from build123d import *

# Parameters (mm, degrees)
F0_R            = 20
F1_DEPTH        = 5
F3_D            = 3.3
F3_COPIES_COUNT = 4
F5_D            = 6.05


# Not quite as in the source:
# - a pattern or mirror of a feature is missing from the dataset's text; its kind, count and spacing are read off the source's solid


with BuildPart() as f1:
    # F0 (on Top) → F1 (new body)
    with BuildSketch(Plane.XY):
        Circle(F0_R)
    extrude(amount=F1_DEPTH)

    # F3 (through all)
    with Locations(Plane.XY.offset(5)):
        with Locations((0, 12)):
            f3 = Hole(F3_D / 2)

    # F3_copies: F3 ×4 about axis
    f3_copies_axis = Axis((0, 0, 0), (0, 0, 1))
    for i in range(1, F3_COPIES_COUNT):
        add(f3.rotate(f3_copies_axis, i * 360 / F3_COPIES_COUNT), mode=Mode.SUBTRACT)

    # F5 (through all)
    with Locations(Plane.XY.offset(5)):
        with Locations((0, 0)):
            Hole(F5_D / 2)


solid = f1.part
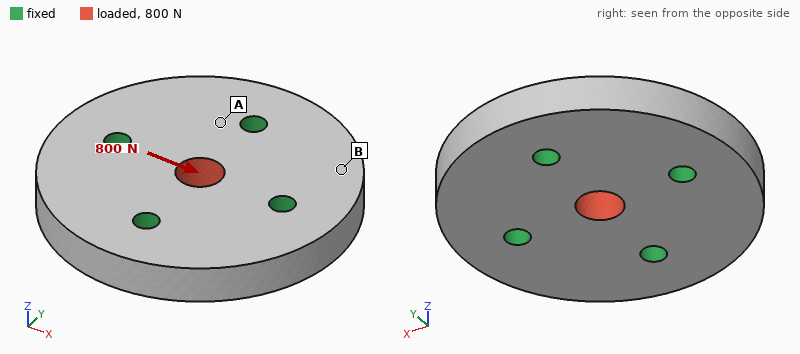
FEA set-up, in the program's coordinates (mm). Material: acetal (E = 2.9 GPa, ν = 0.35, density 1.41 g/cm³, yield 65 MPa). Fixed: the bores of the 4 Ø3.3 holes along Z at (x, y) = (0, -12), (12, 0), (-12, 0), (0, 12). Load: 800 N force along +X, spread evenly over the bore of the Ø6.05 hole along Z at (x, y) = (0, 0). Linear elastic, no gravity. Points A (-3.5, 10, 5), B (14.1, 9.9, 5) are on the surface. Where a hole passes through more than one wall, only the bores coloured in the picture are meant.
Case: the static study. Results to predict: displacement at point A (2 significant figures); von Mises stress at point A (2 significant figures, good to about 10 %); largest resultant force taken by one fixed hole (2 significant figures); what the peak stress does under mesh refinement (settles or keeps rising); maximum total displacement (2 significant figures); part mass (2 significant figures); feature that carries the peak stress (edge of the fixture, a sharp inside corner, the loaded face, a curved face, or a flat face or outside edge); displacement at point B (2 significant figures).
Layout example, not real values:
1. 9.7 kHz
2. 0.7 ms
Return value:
1. 4.3 µm
2. 2.2 MPa
3. 270 N
4. keeps rising
5. 24 µm
6. 8.4 g
7. edge of the fixture
8. 5.8 µm
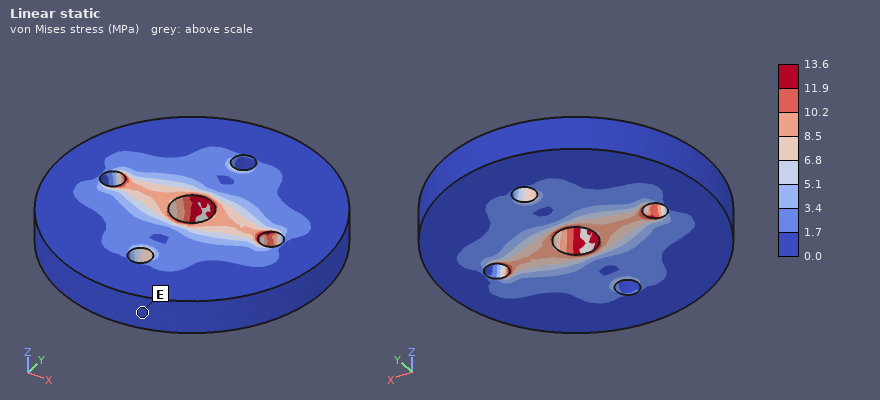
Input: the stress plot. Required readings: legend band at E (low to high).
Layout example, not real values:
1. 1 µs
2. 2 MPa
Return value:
1. 0.0 to 1.7 MPa
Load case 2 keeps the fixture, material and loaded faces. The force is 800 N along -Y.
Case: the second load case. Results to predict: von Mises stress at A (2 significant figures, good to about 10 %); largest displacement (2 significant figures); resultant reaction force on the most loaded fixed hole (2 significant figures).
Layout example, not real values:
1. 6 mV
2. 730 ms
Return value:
1. 3.0 MPa
2. 24 µm
3. 270 N
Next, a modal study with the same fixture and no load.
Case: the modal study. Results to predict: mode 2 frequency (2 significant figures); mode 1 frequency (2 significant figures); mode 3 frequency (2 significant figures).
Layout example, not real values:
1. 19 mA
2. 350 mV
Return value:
1. 9000 Hz
2. 8200 Hz
3. 9000 Hz
